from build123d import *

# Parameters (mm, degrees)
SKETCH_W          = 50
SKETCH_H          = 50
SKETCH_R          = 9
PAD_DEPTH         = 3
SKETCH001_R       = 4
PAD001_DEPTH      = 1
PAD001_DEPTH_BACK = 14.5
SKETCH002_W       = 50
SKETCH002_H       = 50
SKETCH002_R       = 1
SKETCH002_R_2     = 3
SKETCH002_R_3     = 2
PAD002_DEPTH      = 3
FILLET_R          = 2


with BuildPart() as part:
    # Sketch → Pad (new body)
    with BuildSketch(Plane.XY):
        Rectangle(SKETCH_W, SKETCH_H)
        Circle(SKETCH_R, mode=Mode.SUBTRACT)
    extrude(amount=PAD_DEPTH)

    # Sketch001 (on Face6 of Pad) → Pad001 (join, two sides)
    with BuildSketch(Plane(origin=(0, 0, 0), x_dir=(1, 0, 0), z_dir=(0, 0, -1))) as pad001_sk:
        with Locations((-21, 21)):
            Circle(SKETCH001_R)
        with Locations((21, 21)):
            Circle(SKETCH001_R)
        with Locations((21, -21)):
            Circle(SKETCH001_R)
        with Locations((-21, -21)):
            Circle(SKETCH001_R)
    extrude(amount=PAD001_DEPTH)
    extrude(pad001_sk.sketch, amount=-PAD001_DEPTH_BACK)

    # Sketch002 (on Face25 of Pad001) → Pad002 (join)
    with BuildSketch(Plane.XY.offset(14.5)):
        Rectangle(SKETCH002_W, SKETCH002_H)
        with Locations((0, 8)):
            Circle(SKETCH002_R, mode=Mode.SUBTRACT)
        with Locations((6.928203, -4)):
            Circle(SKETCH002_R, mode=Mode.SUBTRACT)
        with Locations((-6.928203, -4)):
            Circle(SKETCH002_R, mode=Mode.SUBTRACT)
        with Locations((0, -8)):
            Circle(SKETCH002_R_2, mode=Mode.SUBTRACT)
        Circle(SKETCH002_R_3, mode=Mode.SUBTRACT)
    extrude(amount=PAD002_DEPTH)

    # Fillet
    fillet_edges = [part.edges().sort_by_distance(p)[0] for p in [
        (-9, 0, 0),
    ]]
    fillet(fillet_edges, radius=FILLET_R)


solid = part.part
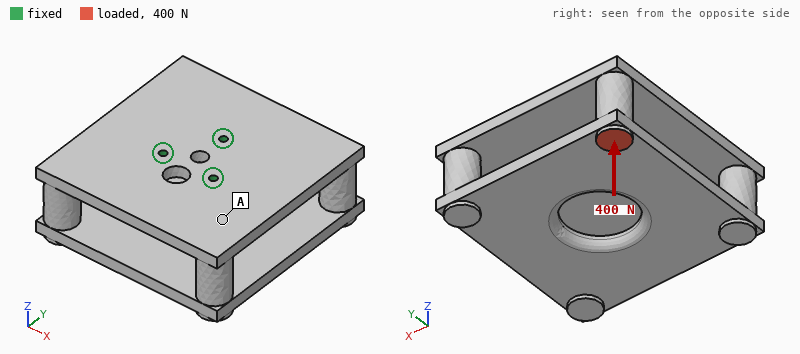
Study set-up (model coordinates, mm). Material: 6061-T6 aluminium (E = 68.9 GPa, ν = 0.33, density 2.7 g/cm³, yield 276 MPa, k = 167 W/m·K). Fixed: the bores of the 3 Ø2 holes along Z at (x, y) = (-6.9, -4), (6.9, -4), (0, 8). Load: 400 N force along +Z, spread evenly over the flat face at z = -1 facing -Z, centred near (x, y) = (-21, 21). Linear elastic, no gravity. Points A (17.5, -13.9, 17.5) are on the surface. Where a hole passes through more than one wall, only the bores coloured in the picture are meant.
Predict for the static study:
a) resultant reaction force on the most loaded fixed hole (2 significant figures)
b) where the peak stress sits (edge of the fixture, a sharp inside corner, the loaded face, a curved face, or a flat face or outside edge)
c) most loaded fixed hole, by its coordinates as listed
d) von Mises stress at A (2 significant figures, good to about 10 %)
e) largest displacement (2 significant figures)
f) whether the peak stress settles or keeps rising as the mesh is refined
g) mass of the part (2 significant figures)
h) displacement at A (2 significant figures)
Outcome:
550 N
edge of the fixture
(0, 8)
15 MPa
0.25 mm
keeps rising
45 g
0.050 mm
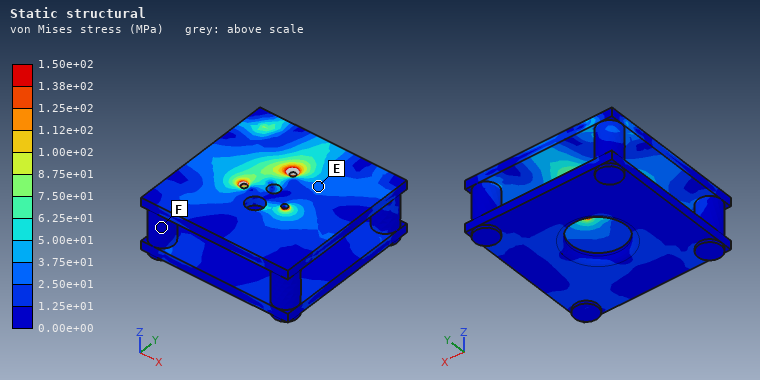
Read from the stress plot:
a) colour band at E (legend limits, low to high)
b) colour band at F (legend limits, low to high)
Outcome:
2.50e+01 to 3.75e+01 MPa
0.00e+00 to 1.25e+01 MPa
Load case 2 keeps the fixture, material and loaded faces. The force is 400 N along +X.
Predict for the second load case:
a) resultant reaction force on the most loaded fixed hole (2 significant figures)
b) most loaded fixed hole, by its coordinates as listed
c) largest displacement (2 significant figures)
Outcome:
490 N
(0, 8)
0.15 mm
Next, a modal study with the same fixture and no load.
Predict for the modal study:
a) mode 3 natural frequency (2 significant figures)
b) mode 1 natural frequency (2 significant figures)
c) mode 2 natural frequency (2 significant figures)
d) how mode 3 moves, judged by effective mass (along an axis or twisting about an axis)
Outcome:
2900 Hz
1900 Hz
1900 Hz
along Z
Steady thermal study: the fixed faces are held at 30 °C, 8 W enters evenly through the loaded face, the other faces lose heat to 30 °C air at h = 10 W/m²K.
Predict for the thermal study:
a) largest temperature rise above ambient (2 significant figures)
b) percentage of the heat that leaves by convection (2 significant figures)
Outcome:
19 K
8.0 %
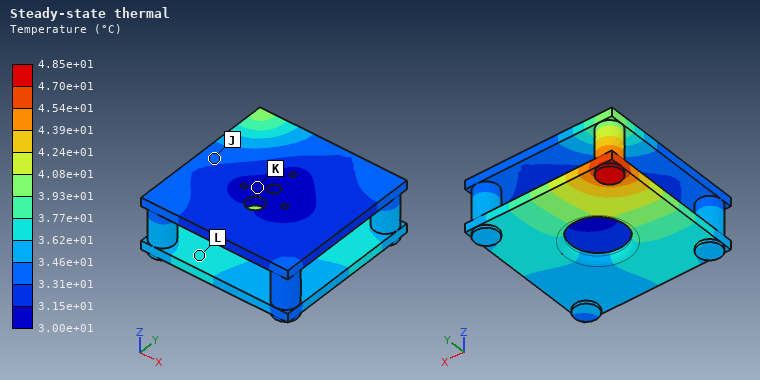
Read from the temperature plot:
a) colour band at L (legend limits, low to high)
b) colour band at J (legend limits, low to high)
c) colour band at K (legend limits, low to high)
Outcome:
3.62e+01 to 3.77e+01 °C
3.31e+01 to 3.46e+01 °C
3.00e+01 to 3.15e+01 °C
